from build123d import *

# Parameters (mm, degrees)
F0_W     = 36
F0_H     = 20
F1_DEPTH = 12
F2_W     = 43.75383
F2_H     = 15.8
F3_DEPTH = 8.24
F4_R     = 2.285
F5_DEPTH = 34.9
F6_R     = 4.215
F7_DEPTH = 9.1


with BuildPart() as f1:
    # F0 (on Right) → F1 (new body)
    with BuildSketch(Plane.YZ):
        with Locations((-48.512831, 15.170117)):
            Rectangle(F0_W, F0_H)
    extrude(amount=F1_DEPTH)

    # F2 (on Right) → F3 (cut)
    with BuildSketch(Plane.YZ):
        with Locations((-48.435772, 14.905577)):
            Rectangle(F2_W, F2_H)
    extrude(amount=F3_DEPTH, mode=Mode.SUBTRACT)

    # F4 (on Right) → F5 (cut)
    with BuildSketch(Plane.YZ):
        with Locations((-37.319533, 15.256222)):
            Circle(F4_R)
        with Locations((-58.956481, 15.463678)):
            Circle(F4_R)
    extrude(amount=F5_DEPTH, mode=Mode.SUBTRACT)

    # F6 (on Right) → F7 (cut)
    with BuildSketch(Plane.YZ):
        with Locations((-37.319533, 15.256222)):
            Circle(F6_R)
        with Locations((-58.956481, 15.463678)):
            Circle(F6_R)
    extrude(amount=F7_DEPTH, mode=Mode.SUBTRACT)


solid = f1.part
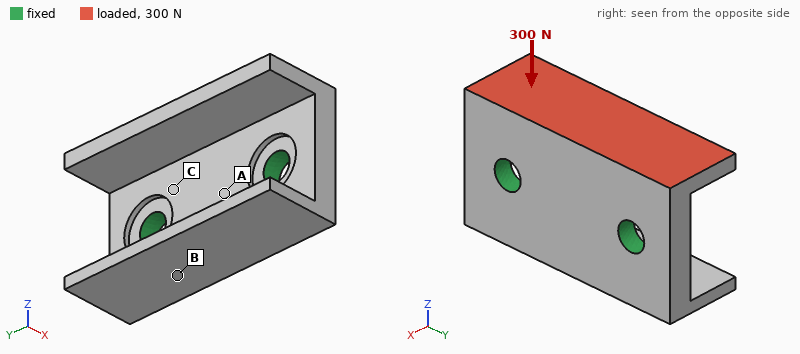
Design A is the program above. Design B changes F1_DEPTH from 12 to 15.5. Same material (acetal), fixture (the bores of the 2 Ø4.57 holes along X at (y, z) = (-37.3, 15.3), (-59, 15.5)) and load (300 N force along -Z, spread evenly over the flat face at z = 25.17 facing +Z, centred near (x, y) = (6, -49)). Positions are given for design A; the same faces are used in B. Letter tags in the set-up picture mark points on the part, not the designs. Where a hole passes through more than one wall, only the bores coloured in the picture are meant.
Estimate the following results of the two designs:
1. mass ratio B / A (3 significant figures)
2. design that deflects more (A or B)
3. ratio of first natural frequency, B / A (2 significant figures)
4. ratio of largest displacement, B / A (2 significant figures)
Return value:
1.64
A
1.5
0.41
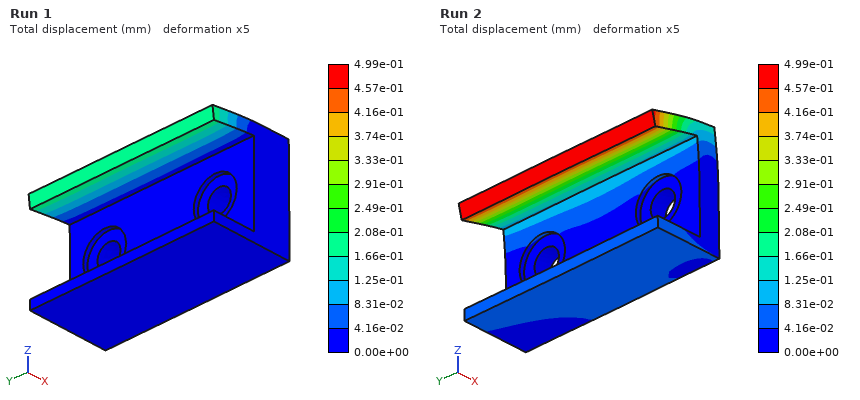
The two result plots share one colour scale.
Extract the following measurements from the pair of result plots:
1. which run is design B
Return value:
Run 1
